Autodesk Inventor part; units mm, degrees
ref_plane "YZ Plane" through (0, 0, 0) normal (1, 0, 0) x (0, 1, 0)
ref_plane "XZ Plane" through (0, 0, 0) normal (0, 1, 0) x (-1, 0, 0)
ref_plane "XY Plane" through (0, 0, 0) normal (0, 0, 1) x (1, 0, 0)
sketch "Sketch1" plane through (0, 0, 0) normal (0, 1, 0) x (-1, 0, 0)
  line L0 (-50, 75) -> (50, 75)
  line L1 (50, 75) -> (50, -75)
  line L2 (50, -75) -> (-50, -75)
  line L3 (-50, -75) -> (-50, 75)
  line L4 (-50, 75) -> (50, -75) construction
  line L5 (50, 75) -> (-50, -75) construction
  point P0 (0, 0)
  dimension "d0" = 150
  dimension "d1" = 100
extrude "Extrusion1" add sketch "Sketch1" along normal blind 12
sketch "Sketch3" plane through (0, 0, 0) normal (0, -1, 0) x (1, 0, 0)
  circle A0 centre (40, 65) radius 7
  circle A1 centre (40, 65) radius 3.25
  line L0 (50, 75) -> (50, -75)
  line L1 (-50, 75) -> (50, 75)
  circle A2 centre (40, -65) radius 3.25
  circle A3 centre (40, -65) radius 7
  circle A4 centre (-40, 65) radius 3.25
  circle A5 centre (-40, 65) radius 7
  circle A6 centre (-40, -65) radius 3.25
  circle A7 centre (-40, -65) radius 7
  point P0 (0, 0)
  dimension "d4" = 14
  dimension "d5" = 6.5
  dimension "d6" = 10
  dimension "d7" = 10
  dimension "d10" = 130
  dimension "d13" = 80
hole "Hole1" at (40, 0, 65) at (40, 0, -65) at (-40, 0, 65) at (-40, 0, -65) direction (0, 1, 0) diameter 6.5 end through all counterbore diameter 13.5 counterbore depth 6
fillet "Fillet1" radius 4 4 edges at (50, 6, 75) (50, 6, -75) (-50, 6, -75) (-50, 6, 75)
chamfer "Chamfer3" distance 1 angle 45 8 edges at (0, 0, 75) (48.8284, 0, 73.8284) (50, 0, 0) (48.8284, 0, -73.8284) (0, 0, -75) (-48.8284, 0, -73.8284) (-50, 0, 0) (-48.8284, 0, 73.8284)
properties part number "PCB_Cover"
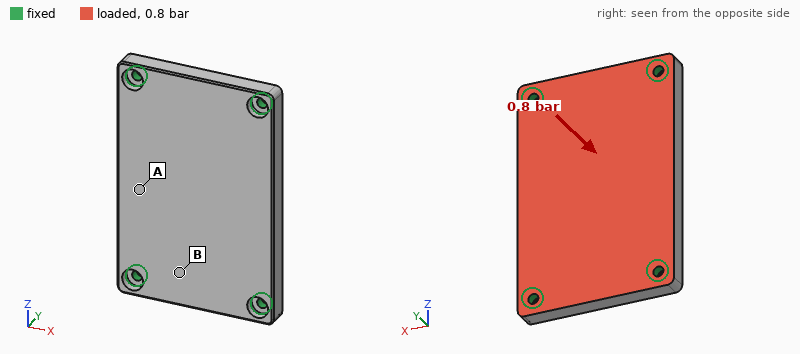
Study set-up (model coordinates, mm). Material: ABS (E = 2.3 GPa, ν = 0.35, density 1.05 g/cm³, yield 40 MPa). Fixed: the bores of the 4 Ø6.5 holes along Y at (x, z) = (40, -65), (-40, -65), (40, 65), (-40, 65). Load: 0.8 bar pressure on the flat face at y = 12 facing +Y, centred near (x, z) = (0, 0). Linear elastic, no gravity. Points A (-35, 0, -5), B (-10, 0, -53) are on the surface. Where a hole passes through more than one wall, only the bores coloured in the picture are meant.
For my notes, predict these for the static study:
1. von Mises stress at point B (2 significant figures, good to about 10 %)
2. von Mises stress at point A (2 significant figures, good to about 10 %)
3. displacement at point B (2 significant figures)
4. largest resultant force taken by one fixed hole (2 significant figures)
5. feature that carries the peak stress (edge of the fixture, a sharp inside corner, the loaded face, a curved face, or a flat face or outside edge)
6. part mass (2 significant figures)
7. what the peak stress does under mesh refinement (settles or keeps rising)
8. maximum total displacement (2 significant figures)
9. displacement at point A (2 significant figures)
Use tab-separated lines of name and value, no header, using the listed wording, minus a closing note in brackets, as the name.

von Mises stress at point B	1.7 MPa
von Mises stress at point A	4.1 MPa
displacement at point B	0.17 mm
largest resultant force taken by one fixed hole	420 N
feature that carries the peak stress	edge of the fixture
part mass	180 g
what the peak stress does under mesh refinement	keeps rising
maximum total displacement	0.43 mm
displacement at point A	0.41 mm
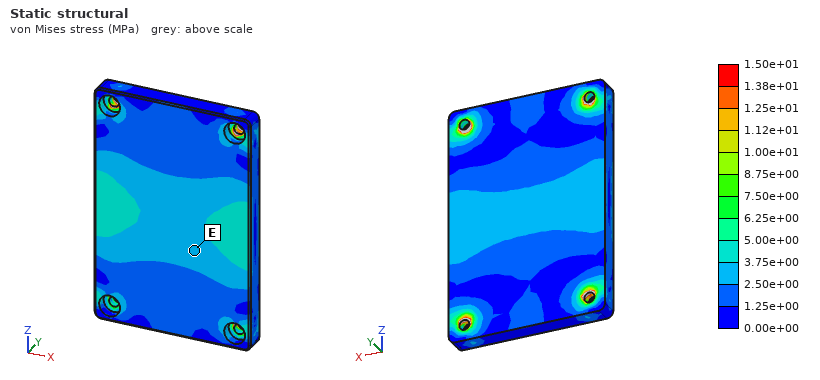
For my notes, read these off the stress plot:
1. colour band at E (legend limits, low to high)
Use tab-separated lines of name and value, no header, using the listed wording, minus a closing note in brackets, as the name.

colour band at E	2.50e+00 to 3.75e+00 MPa
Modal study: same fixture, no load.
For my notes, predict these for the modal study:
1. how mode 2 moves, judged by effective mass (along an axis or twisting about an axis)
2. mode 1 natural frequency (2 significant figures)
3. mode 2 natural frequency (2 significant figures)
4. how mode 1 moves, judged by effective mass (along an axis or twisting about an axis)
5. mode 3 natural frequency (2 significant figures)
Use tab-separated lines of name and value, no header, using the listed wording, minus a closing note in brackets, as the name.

how mode 2 moves, judged by effective mass	twisting about Z
mode 1 natural frequency	690 Hz
mode 2 natural frequency	1100 Hz
how mode 1 moves, judged by effective mass	along Y
mode 3 natural frequency	1700 Hz
